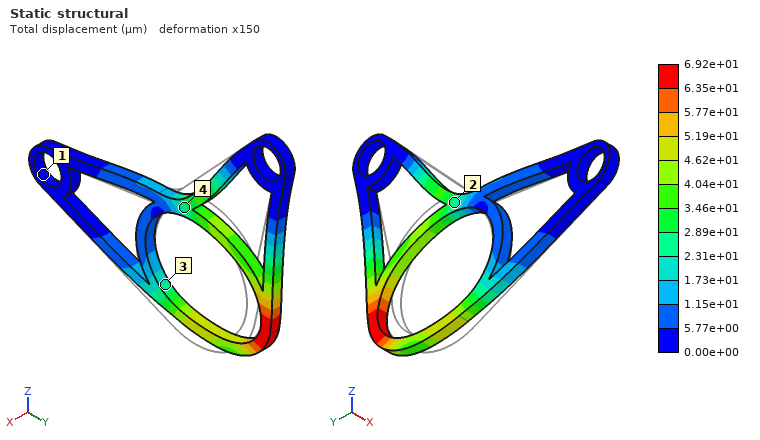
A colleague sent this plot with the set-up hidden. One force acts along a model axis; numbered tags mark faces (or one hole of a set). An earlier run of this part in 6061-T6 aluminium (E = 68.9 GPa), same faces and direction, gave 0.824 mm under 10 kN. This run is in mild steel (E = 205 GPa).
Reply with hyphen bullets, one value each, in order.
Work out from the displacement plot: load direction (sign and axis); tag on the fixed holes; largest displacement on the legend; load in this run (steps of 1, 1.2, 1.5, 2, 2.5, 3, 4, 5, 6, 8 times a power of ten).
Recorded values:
- +Y
- 1
- 6.92e+01 µm
- 2.5 kN
